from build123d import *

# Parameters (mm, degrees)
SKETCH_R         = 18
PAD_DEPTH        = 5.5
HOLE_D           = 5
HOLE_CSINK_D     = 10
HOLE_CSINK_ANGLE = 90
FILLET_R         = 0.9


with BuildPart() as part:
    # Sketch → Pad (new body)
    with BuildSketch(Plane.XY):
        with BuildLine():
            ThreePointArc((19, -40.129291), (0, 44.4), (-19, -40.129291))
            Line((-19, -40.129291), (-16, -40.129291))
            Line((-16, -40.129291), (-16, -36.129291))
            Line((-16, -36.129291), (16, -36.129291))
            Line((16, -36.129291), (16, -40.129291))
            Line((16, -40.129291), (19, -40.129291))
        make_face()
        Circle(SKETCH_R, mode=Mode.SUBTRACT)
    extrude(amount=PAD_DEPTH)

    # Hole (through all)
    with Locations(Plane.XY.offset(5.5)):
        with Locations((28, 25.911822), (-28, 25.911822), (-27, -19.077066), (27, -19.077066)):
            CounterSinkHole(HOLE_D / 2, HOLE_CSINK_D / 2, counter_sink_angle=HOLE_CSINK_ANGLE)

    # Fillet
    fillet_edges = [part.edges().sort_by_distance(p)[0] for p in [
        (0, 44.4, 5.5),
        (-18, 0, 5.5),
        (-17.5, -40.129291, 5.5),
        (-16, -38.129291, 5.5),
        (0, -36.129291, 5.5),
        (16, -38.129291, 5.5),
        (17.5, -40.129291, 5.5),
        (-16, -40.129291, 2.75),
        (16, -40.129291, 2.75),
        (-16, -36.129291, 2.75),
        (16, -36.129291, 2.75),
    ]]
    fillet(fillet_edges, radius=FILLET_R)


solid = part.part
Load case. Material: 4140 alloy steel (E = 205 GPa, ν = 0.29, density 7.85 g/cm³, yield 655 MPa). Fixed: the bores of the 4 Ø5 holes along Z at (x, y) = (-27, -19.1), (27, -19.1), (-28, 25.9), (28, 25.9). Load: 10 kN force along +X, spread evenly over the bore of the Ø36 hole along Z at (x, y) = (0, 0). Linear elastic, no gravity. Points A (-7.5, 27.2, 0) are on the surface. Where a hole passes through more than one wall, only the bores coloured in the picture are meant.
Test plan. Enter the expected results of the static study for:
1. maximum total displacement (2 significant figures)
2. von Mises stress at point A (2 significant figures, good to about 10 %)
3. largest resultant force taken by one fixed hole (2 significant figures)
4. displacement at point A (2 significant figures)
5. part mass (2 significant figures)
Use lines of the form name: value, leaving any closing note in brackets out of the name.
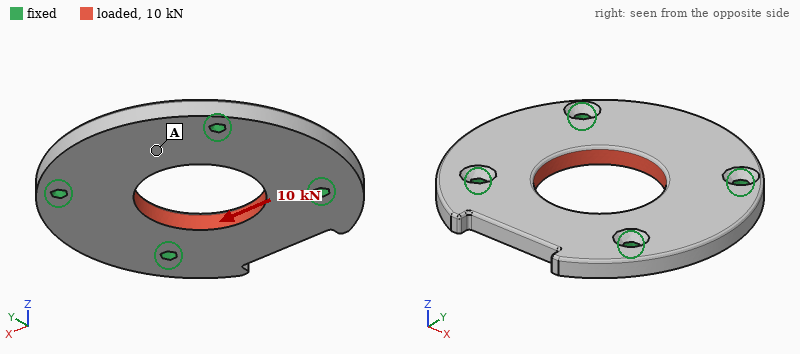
maximum total displacement: 3.9 µm
von Mises stress at point A: 14 MPa
largest resultant force taken by one fixed hole: 2.7 kN
displacement at point A: 1.9 µm
part mass: 210 g
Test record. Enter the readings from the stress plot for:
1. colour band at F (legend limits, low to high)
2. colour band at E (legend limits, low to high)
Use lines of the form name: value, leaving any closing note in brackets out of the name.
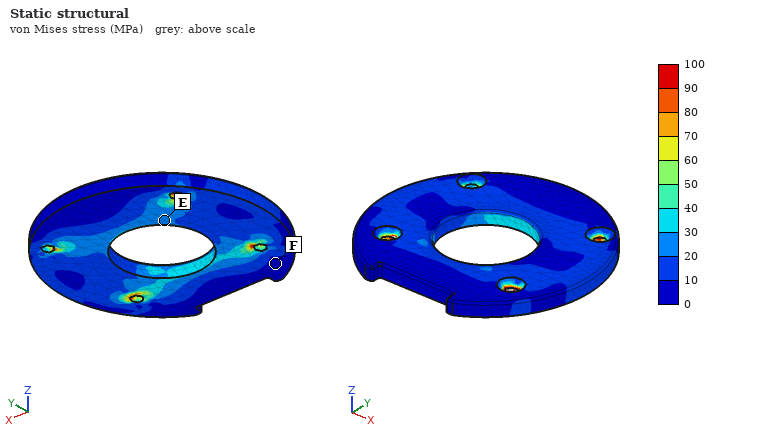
colour band at F: 0 to 10 MPa
colour band at E: 20 to 30 MPa
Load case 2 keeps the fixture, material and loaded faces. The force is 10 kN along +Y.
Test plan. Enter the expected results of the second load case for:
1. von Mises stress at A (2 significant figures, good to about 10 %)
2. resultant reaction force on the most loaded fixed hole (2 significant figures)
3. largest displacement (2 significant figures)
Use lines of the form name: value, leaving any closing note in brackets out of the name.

von Mises stress at A: 16 MPa
resultant reaction force on the most loaded fixed hole: 2.8 kN
largest displacement: 6.2 µm
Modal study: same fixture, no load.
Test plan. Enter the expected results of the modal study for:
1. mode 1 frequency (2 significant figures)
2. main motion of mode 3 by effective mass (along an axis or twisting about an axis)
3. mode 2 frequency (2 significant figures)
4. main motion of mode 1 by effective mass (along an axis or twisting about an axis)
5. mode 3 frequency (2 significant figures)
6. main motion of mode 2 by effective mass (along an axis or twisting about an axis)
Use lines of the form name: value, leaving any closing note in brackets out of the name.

mode 1 frequency: 6200 Hz
main motion of mode 3 by effective mass: twisting about Y
mode 2 frequency: 6600 Hz
main motion of mode 1 by effective mass: along Z
mode 3 frequency: 9000 Hz
main motion of mode 2 by effective mass: twisting about X
